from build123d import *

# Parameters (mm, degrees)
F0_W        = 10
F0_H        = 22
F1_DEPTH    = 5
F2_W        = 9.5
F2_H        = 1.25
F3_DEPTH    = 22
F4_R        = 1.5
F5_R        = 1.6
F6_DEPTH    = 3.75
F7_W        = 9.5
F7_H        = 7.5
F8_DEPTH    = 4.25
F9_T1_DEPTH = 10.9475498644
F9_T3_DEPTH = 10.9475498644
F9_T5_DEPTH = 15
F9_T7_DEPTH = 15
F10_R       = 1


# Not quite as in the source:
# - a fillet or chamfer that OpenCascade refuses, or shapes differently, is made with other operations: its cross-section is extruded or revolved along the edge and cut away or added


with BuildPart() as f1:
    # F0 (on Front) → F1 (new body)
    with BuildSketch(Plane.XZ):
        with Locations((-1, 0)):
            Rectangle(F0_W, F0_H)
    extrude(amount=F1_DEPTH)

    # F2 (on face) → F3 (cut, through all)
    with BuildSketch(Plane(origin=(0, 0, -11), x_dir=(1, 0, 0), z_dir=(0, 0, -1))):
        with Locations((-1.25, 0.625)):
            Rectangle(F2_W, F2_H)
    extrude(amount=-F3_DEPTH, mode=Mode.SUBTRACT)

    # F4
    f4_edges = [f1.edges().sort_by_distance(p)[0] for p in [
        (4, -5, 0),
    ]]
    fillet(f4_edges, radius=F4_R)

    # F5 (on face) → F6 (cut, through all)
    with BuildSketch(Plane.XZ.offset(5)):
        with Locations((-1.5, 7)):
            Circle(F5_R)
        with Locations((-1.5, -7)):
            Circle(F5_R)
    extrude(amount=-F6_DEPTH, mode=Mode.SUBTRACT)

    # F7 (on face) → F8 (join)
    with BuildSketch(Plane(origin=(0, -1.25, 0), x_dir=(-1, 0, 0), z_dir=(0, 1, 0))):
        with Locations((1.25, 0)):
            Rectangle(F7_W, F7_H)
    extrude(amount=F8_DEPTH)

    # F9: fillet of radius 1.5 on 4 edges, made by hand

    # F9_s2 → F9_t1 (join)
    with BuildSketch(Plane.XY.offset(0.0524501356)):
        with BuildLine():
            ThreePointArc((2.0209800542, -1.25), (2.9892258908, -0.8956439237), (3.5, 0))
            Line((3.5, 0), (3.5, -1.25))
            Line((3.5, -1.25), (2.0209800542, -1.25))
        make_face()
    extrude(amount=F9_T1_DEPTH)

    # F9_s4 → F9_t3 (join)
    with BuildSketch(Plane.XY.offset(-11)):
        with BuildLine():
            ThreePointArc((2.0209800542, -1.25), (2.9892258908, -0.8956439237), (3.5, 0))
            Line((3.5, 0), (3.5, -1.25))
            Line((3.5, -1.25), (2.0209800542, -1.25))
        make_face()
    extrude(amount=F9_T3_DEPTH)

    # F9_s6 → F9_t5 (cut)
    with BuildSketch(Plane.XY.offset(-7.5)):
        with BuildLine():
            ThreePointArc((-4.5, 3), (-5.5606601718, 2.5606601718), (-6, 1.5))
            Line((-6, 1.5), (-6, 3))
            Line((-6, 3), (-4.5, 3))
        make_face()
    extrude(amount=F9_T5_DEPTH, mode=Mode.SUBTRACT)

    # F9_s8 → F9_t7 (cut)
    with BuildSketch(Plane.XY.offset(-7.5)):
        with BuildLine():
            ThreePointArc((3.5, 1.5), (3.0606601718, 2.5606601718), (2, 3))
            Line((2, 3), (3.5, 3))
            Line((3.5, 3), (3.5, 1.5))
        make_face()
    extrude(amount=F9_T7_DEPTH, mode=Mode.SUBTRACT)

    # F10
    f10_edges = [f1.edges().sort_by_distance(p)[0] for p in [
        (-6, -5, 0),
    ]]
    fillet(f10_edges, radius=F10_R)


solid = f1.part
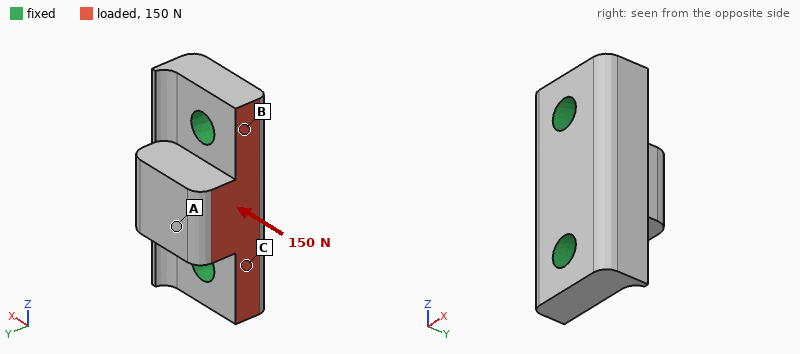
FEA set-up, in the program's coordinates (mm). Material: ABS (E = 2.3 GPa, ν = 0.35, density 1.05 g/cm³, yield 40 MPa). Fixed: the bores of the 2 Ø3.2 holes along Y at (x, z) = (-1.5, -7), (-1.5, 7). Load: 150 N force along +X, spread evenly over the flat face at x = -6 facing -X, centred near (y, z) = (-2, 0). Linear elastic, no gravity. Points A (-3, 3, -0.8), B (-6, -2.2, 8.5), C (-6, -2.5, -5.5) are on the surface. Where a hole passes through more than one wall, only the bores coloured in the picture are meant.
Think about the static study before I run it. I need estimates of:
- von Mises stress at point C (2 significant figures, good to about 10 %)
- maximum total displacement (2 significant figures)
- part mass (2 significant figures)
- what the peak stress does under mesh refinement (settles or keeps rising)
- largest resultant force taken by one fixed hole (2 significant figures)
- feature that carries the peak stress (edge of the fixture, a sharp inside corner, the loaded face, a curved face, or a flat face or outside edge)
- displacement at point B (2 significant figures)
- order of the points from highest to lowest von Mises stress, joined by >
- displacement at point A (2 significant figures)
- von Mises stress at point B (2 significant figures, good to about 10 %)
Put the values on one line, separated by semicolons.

2.9 MPa; 23 µm; 1.1 g; keeps rising; 75 N; edge of the fixture; 4.0 µm; C > B > A; 22 µm; 2.2 MPa
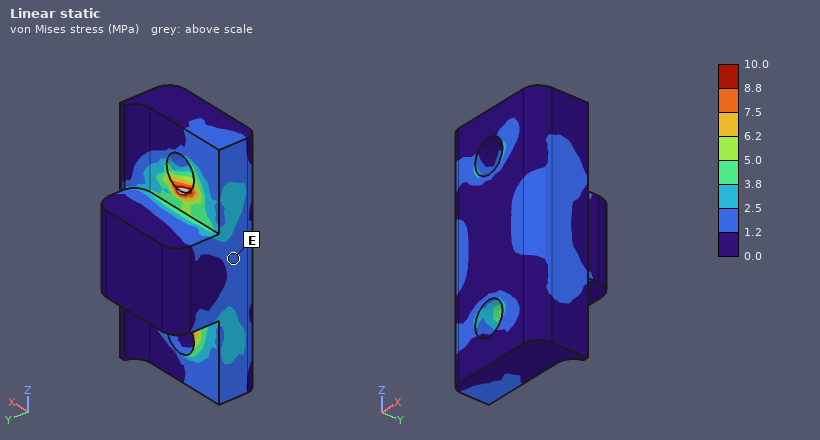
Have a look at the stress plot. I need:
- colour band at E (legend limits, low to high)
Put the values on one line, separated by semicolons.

1.2 to 2.5 MPa
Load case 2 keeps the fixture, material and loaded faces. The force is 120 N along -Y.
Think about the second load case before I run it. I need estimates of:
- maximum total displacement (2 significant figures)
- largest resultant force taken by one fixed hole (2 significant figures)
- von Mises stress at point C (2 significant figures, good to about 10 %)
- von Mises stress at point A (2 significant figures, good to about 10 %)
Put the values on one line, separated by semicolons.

41 µm; 61 N; 5.5 MPa; 1.5 MPa
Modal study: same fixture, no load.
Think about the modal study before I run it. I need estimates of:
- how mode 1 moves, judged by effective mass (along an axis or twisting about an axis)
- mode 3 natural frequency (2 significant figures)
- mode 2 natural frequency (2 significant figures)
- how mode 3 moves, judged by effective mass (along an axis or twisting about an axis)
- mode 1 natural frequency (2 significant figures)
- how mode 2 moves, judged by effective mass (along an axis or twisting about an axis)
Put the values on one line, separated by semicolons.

along X; 23 kHz; 19 kHz; along Z; 12 kHz; along Y
